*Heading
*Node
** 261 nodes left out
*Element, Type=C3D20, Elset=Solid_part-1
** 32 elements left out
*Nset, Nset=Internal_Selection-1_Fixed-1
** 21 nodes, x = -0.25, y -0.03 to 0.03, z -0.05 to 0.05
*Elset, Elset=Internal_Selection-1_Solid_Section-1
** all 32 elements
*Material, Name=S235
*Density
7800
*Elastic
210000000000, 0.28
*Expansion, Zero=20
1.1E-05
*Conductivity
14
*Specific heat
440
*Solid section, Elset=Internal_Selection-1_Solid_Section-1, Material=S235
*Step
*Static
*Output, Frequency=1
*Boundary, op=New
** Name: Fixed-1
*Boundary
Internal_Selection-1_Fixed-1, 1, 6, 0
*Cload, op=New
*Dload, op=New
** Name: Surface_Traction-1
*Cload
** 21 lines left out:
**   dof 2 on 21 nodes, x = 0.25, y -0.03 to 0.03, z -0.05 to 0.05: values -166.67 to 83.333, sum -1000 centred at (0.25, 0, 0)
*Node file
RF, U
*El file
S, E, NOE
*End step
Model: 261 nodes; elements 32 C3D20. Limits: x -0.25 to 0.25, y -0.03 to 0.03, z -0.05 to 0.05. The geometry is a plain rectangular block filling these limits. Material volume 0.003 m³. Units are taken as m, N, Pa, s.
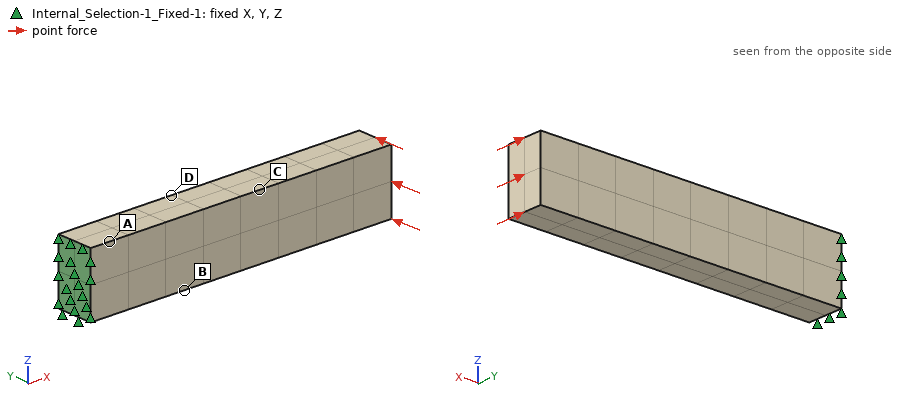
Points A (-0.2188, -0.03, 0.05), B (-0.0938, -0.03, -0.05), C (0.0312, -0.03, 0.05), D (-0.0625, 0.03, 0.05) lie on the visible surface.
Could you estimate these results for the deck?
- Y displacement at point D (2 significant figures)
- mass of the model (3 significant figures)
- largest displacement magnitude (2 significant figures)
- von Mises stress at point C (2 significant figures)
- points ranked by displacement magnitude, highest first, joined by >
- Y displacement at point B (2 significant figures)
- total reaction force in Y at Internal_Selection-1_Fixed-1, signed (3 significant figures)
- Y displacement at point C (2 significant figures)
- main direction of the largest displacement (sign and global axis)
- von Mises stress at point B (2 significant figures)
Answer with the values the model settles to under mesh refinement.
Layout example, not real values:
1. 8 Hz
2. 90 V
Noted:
1. -2.0e-05 m
2. 23.4 kg
3. 1.1e-04 m
4. 3.6e+06 Pa
5. C > D > B > A
6. -1.4e-05 m
7. 1000 N
8. -4.2e-05 m
9. -Y
10. 5.7e+06 Pa
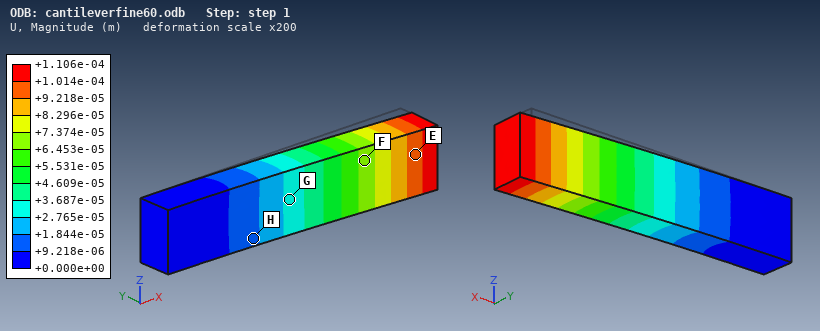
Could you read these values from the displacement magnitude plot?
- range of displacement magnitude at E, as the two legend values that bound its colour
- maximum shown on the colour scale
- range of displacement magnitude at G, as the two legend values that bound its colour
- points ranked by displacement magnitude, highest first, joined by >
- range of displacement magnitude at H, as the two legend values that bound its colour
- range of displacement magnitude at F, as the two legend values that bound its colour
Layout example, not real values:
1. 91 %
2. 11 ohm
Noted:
1. +9.218e-05 to +1.014e-04 m
2. +1.106e-04 m
3. +2.765e-05 to +3.687e-05 m
4. E > F > G > H
5. +9.218e-06 to +1.844e-05 m
6. +6.453e-05 to +7.374e-05 m
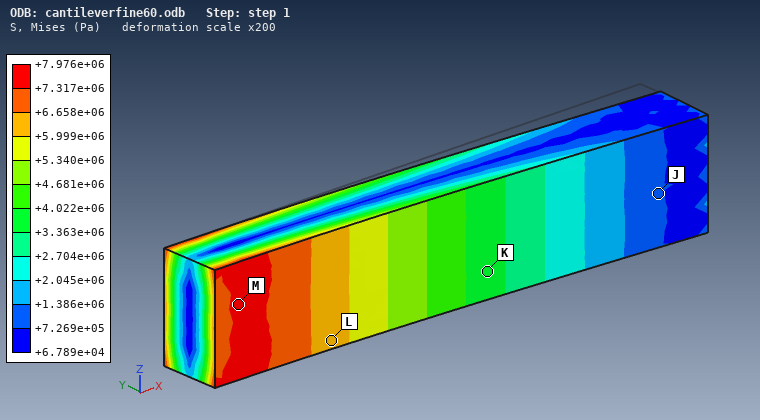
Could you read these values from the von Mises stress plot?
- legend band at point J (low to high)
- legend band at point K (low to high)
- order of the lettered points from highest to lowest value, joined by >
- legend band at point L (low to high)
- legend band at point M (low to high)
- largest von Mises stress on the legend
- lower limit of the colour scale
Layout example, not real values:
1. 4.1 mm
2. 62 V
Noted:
1. +7.269e+05 to +1.386e+06 Pa
2. +3.363e+06 to +4.022e+06 Pa
3. M > L > K > J
4. +5.999e+06 to +6.658e+06 Pa
5. +7.317e+06 to +7.976e+06 Pa
6. +7.976e+06 Pa
7. +6.789e+04 Pa
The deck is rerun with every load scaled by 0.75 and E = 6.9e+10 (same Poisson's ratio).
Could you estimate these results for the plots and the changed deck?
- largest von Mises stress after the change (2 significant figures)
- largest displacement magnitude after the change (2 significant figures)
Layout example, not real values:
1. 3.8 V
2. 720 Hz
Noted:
1. 6.0e+06 Pa
2. 2.5e-04 m
